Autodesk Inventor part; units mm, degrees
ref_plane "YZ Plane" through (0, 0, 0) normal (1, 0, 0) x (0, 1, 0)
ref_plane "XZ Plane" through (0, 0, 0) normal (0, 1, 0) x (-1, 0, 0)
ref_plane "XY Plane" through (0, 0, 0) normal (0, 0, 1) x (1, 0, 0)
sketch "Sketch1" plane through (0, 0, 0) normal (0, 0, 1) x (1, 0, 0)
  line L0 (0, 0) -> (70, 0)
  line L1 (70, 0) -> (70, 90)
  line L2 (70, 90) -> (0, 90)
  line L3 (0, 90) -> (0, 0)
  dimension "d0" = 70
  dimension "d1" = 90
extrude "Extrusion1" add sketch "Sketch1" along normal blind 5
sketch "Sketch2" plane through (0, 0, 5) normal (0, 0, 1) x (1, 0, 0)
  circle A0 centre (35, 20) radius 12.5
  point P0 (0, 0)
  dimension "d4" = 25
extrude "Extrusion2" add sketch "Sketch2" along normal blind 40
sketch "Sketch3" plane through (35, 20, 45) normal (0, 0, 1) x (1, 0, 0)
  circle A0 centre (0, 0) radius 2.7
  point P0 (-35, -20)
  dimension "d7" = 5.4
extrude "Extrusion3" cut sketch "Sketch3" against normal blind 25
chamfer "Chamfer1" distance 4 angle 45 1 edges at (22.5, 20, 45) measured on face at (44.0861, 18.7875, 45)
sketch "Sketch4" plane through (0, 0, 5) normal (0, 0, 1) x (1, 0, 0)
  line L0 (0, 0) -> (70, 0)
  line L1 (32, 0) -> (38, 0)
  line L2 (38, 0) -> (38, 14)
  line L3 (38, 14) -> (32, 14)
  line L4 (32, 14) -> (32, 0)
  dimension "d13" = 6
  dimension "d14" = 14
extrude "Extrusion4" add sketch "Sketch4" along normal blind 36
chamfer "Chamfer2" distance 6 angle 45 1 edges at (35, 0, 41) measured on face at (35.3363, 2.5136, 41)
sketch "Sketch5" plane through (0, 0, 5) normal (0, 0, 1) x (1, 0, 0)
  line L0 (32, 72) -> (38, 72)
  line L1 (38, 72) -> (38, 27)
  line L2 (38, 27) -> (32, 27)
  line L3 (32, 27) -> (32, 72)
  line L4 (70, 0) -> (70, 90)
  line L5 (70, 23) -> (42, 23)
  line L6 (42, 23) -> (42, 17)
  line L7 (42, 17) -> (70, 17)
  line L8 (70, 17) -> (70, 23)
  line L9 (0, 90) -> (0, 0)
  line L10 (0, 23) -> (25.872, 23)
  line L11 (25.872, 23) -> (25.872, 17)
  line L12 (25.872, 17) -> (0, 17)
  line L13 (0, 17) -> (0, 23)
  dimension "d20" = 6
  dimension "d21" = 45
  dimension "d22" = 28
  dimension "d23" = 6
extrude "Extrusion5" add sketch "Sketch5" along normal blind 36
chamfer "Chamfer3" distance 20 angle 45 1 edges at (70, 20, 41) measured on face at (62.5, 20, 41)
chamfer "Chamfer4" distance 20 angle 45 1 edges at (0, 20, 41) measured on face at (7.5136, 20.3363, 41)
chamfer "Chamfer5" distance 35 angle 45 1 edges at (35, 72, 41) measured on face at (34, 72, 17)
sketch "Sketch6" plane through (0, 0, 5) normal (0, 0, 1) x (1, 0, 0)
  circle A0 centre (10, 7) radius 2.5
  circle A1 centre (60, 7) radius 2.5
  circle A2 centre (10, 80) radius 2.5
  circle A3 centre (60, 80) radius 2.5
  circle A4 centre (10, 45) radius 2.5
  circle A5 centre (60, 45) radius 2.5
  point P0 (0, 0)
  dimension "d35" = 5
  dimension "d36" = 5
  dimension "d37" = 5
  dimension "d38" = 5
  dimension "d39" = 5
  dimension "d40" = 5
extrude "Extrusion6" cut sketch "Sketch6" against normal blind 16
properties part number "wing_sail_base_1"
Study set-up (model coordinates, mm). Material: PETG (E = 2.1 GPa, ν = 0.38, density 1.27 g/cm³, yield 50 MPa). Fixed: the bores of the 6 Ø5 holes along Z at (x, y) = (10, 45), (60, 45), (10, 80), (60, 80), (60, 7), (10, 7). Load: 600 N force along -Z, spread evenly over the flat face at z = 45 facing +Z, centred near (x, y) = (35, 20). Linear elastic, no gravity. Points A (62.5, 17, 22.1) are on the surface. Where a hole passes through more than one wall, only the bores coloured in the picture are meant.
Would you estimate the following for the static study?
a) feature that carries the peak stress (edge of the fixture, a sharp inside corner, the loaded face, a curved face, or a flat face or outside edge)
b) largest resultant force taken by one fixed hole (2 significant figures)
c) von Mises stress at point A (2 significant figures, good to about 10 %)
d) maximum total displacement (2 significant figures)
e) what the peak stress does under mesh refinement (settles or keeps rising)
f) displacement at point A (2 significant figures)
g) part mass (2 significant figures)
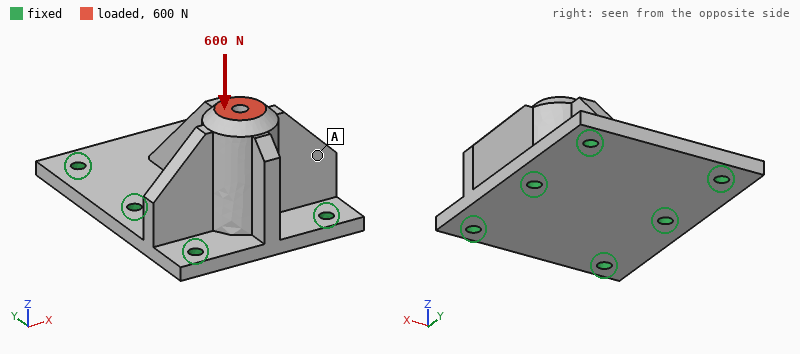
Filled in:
edge of the fixture
220 N
1.6 MPa
0.15 mm
keeps rising
0.093 mm
80 g
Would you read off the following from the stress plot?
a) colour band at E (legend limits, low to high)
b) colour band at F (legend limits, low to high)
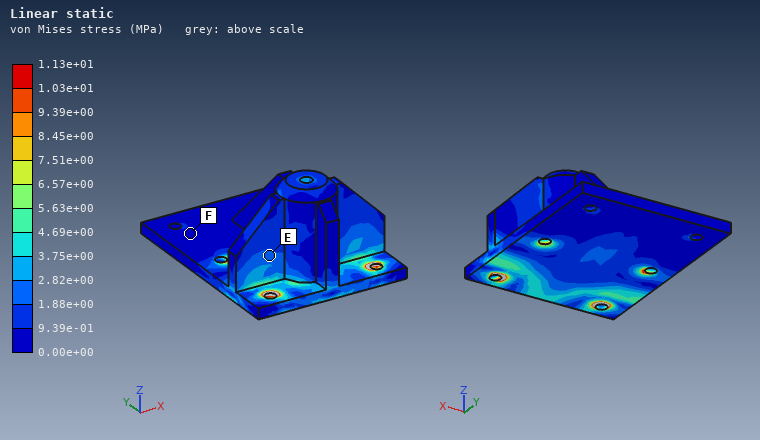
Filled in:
1.88e+00 to 2.82e+00 MPa
0.00e+00 to 9.39e-01 MPa
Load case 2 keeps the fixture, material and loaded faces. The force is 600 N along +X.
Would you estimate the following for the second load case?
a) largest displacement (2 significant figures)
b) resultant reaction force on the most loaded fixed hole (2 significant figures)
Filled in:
0.44 mm
430 N
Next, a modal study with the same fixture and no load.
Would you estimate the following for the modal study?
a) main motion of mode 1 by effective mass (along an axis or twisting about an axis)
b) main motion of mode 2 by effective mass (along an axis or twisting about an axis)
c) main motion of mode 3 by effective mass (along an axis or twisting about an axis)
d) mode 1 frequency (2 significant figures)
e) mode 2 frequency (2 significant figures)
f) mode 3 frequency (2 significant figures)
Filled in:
along Y
along X
along Z
1300 Hz
1600 Hz
1700 Hz
